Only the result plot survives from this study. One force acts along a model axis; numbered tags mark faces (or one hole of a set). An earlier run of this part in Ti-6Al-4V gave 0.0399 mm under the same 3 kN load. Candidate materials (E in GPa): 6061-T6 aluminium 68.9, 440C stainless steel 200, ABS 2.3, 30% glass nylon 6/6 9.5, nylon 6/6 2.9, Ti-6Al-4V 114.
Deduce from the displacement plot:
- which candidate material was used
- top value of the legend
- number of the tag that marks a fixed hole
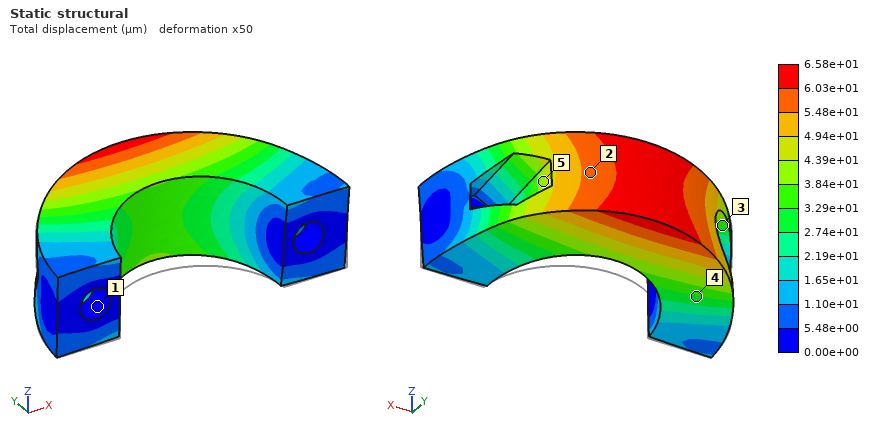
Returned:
6061-T6 aluminium
6.58e+01 µm
1
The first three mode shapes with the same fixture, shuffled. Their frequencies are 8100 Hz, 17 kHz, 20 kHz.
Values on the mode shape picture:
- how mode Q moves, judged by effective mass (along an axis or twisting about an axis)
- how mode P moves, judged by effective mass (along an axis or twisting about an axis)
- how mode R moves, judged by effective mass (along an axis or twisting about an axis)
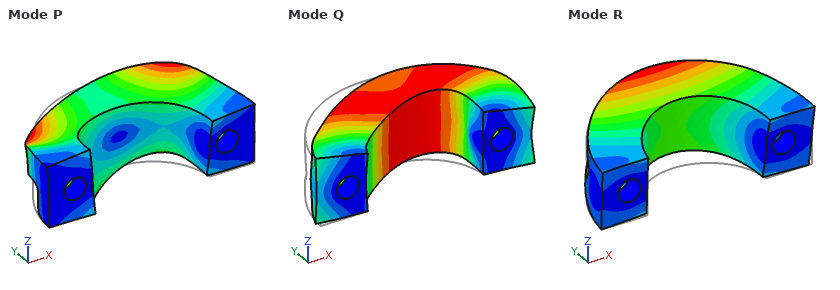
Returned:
along X
twisting about Y
along Z
